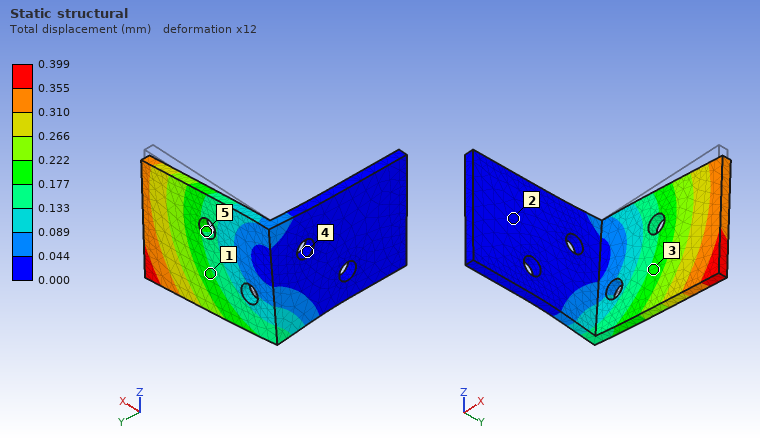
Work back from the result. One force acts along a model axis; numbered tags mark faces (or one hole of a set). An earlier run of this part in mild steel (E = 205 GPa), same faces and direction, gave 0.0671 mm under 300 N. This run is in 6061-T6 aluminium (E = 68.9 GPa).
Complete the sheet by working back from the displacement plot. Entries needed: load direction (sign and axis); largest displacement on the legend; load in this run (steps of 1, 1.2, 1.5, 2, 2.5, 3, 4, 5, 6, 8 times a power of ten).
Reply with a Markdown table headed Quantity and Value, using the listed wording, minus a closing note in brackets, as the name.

| Quantity | Value |
|---|---|
| load direction | -Z |
| largest displacement on the legend | 0.399 mm |
| load in this run | 600 N |
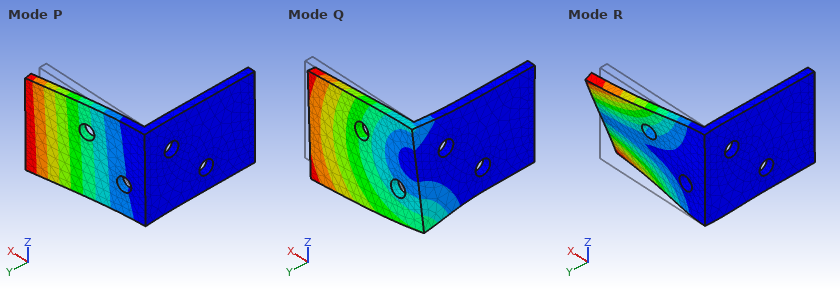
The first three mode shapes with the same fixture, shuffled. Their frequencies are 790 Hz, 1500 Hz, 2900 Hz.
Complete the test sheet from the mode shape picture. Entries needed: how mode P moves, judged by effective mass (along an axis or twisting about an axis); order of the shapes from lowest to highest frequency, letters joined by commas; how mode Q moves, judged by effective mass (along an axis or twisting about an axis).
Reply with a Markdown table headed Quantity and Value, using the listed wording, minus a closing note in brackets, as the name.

| Quantity | Value |
|---|---|
| how mode P moves, judged by effective mass | along Y |
| order of the shapes from lowest to highest frequency, letters joined by commas | P, Q, R |
| how mode Q moves, judged by effective mass | along Z |
